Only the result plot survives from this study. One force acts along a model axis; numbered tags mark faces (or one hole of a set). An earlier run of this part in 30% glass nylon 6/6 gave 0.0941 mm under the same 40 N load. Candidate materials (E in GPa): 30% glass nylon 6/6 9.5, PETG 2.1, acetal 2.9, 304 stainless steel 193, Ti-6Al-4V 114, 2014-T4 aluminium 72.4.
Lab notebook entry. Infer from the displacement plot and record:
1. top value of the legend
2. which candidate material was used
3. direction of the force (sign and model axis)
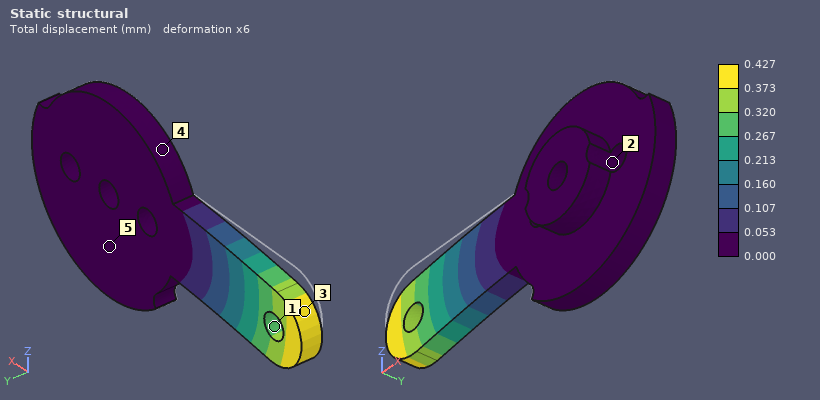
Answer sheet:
0.427 mm
PETG
-Z
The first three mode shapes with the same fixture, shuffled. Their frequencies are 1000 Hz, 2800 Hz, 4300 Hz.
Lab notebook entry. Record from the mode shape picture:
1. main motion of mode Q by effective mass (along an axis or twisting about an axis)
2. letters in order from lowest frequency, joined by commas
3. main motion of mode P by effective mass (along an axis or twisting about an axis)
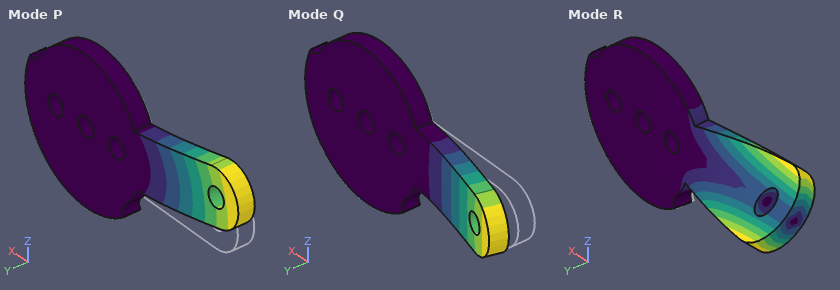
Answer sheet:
along Y
Q, P, R
along Z
